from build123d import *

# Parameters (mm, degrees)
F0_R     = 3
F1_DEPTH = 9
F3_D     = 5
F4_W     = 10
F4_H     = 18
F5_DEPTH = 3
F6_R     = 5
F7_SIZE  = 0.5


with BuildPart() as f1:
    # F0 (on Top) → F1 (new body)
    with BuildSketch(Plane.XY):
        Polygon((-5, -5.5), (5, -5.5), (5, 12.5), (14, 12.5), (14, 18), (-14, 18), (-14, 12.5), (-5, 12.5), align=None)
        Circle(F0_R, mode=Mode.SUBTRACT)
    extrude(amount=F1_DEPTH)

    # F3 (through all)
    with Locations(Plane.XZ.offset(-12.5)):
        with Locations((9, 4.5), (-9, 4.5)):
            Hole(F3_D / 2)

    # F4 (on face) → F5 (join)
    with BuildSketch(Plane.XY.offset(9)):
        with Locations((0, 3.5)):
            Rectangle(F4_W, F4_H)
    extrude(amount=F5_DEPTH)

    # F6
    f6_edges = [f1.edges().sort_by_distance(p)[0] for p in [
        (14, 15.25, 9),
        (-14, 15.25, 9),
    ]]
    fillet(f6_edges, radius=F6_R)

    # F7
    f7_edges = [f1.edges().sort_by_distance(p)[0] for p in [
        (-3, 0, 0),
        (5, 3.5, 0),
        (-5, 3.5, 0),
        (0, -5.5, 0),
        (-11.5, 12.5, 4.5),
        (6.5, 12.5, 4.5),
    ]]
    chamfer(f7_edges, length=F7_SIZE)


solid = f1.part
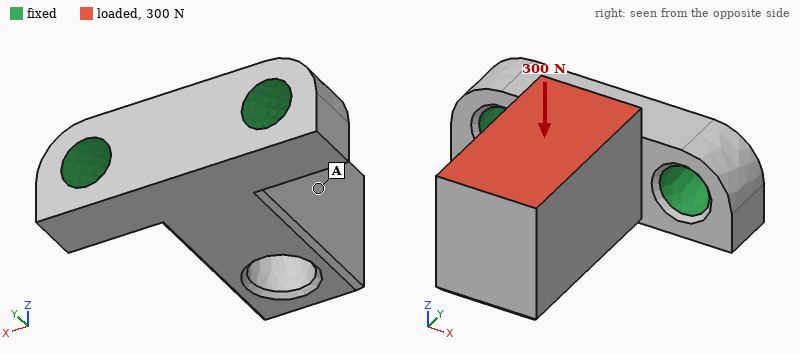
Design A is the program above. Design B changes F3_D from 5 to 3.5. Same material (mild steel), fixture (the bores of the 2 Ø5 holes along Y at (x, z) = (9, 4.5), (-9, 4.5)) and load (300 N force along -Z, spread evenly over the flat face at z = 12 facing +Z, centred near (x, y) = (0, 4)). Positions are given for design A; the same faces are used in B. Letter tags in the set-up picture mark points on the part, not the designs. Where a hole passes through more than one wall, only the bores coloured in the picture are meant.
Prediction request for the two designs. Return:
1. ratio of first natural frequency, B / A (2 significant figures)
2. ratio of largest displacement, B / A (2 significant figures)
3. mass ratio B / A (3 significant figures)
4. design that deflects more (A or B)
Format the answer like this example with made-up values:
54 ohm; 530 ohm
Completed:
0.91; 1.2; 1.04; B
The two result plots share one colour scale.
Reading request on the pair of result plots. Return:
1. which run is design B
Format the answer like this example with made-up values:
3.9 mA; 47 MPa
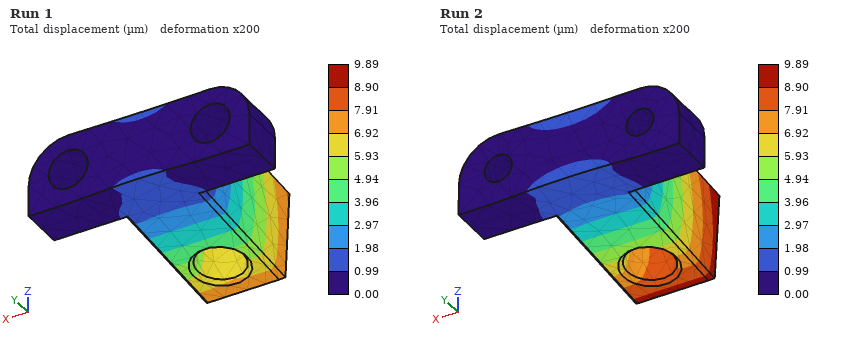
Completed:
Run 2
